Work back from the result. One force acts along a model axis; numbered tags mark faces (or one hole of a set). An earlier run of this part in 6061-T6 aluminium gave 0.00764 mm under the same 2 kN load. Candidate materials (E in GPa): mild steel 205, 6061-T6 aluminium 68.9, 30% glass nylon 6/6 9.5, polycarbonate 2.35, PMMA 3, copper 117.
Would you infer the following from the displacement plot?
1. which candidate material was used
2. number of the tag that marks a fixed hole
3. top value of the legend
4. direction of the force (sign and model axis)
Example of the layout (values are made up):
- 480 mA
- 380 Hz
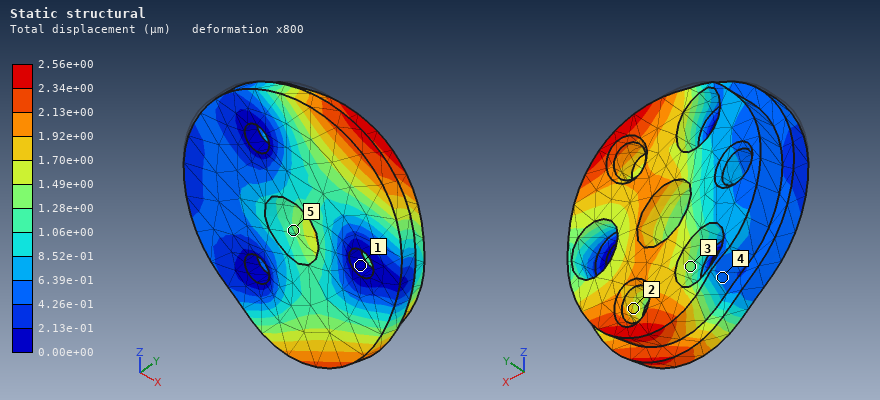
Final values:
- mild steel
- 1
- 2.56e+00 µm
- -Z
